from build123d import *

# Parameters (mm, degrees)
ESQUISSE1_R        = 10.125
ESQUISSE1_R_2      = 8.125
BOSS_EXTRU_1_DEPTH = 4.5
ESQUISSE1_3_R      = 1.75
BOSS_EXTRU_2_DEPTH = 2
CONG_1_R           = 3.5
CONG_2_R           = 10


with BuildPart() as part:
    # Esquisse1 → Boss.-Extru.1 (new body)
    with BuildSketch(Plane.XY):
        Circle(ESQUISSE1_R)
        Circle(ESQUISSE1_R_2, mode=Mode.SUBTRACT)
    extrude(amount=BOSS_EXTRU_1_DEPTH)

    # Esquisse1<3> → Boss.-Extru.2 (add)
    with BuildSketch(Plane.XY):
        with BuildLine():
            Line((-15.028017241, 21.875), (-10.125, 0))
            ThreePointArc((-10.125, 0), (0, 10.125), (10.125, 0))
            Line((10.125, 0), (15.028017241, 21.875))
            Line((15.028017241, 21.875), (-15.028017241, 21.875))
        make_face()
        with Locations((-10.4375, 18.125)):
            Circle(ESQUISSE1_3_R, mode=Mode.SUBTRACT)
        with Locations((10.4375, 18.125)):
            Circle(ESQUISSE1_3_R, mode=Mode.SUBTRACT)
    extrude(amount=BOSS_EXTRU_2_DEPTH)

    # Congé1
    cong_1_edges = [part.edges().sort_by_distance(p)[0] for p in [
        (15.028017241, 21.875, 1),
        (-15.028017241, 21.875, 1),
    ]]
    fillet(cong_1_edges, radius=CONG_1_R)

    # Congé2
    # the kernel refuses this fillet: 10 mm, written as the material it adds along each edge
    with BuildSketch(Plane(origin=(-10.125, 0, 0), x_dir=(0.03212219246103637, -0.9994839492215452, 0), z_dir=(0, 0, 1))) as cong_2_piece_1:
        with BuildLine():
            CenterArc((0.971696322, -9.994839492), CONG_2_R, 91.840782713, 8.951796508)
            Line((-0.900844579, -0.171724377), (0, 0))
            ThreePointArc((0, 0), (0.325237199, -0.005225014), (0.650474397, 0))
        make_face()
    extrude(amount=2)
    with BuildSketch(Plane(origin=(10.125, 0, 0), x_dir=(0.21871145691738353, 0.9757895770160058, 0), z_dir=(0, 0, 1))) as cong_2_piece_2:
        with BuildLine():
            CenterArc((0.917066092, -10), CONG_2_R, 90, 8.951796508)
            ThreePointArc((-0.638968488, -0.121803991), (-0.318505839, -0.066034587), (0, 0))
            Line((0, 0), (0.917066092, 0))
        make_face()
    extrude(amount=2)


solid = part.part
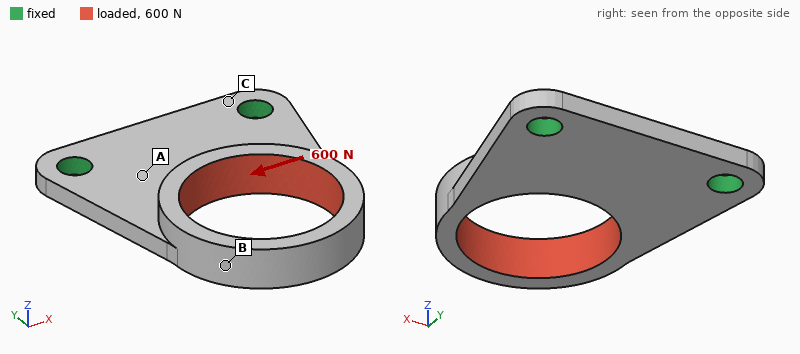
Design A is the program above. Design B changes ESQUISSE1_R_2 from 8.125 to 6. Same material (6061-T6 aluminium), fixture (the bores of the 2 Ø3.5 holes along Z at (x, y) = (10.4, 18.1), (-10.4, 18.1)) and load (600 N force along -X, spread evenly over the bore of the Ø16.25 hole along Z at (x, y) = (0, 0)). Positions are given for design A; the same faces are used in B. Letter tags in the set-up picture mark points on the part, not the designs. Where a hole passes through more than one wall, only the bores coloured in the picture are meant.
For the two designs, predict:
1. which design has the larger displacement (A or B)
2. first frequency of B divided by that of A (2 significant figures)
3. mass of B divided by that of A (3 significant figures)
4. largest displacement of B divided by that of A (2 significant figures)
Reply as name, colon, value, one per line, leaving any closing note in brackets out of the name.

which design has the larger displacement: A
first frequency of B divided by that of A: 0.82
mass of B divided by that of A: 1.34
largest displacement of B divided by that of A: 0.29
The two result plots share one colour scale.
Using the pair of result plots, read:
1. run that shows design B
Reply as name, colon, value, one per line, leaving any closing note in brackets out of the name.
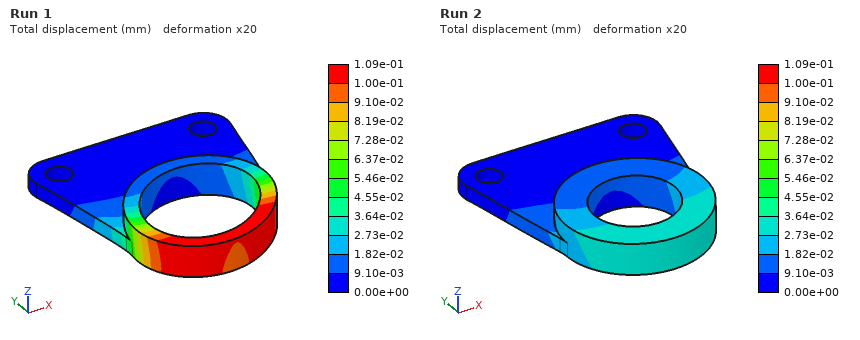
run that shows design B: Run 2
